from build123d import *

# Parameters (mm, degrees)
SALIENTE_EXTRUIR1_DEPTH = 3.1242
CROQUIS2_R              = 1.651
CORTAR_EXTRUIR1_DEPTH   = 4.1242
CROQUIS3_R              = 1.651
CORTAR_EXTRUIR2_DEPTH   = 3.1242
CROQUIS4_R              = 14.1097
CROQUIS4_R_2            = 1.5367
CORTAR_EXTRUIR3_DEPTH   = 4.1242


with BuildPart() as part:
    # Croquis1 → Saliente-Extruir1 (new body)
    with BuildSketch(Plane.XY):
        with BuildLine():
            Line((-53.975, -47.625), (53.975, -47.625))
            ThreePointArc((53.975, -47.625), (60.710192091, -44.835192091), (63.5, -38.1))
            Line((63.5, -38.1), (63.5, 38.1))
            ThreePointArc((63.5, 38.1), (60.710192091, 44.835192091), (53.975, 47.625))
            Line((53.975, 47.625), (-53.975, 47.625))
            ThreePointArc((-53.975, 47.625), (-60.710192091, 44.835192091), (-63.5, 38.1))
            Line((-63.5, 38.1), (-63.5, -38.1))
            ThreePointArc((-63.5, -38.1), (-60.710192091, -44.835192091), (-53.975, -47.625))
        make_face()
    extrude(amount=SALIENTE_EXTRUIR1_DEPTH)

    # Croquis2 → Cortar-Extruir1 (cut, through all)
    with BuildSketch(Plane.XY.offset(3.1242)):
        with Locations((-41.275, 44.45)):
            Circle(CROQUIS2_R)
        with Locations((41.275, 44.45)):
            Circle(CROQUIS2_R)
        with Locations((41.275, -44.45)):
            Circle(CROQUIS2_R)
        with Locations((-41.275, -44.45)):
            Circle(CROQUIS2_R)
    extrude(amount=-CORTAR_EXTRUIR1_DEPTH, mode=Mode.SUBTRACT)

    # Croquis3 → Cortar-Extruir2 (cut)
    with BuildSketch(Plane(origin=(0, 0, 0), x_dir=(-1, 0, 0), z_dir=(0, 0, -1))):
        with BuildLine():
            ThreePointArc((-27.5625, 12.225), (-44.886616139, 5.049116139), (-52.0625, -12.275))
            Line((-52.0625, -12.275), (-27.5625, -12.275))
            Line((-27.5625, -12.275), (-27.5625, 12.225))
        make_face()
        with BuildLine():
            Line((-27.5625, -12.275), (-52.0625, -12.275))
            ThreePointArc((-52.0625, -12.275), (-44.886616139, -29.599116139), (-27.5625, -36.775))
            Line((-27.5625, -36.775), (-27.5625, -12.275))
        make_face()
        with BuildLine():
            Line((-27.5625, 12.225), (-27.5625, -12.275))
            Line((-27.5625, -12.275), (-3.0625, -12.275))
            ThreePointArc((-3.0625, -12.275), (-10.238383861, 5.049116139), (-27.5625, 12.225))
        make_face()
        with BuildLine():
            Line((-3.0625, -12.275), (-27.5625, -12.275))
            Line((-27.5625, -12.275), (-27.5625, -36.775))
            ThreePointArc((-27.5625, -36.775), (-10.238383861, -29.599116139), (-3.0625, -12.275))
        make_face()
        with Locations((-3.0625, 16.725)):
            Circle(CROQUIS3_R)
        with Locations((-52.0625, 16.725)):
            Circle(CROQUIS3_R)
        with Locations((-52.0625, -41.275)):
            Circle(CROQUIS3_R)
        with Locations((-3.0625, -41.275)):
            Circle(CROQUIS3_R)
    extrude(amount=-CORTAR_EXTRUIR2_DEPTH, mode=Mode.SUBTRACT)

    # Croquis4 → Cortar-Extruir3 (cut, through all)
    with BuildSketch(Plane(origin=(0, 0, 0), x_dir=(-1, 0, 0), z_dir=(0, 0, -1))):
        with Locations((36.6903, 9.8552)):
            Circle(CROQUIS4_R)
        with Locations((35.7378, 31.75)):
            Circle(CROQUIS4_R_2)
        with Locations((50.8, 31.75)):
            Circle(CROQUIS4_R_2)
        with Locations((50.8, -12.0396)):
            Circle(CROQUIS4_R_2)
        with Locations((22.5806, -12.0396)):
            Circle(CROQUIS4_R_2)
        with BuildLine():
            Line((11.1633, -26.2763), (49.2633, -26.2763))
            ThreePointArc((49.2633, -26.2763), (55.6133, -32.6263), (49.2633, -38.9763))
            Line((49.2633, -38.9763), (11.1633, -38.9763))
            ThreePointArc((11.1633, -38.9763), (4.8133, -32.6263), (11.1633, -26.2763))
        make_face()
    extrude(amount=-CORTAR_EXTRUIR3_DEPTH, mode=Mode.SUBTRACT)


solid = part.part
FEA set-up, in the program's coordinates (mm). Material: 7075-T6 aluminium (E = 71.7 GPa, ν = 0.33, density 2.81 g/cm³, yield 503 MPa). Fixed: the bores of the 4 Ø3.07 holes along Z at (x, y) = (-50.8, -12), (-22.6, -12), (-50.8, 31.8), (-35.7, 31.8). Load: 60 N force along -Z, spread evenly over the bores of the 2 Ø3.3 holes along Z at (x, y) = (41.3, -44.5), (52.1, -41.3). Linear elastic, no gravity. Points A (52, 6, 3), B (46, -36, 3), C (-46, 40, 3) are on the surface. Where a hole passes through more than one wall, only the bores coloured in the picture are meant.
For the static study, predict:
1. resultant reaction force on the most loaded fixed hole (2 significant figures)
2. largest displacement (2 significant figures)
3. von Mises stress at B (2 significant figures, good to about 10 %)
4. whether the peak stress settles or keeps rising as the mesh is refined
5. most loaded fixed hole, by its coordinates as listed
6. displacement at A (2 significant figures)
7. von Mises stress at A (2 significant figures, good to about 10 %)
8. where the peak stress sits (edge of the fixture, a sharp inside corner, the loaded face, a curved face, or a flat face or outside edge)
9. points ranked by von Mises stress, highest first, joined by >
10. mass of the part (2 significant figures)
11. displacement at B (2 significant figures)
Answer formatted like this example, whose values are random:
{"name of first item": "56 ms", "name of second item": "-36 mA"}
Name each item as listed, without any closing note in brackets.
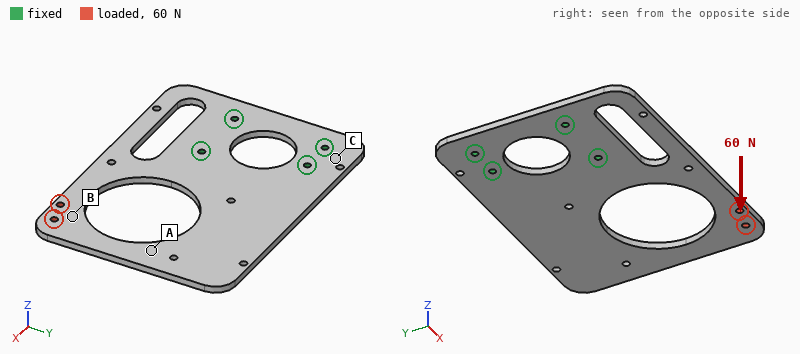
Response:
{"resultant reaction force on the most loaded fixed hole": "140 N", "largest displacement": "1.5 mm", "von Mises stress at B": "17 MPa", "whether the peak stress settles or keeps rising as the mesh is refined": "keeps rising", "most loaded fixed hole, by its coordinates as listed": "(-22.6, -12)", "displacement at A": "0.68 mm", "von Mises stress at A": "28 MPa", "where the peak stress sits": "edge of the fixture", "points ranked by von Mises stress, highest first, joined by >": "A > B > C", "mass of the part": "77 g", "displacement at B": "1.1 mm"}
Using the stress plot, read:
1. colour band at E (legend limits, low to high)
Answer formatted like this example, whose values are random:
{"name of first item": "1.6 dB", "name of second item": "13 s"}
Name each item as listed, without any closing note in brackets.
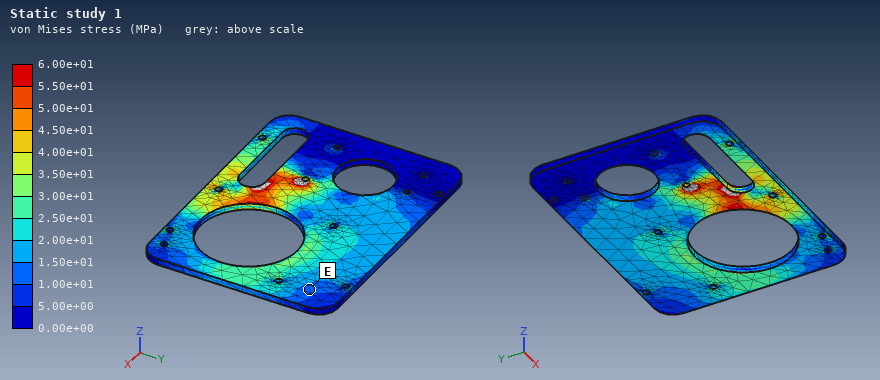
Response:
{"colour band at E": "1.00e+01 to 1.50e+01 MPa"}
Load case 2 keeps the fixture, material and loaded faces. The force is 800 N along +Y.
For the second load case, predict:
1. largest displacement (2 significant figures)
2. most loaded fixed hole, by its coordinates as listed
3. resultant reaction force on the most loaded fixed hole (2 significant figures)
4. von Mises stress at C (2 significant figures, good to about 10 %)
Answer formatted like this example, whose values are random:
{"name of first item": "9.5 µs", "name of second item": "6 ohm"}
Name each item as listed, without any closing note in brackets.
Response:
{"largest displacement": "87 µm", "most loaded fixed hole, by its coordinates as listed": "(-22.6, -12)", "resultant reaction force on the most loaded fixed hole": "1.2 kN", "von Mises stress at C": "9.6 MPa"}
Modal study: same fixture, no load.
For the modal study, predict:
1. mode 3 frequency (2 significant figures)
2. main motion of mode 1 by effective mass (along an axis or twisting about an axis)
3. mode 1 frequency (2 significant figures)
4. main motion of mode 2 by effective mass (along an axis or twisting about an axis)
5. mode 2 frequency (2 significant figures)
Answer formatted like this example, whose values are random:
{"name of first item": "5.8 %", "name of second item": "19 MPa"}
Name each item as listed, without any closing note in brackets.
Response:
{"mode 3 frequency": "1300 Hz", "main motion of mode 1 by effective mass": "along Z", "mode 1 frequency": "280 Hz", "main motion of mode 2 by effective mass": "twisting about X", "mode 2 frequency": "560 Hz"}
